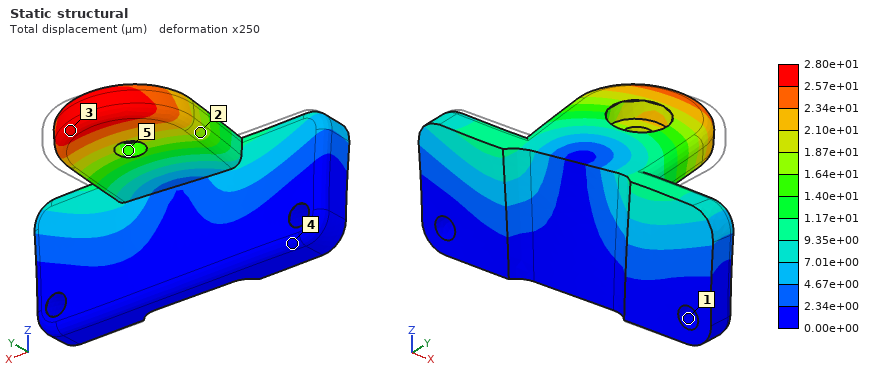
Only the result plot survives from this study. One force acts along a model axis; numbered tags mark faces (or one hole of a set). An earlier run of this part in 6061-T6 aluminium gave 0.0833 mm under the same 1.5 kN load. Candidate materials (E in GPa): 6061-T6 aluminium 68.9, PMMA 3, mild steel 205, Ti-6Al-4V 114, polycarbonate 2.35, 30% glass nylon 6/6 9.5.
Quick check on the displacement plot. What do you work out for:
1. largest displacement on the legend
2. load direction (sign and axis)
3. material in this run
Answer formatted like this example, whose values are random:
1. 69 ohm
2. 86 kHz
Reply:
1. 2.80e+01 µm
2. -X
3. mild steel
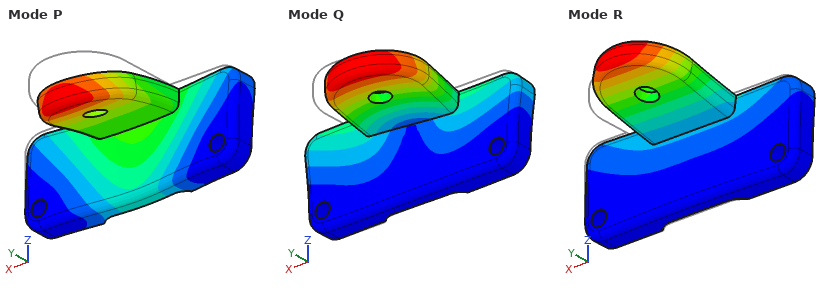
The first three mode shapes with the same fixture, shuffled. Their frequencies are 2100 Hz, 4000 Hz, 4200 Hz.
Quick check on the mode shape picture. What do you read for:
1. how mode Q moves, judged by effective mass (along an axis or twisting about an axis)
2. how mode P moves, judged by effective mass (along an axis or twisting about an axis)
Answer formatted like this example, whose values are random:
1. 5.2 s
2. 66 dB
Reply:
1. along X
2. along Y
